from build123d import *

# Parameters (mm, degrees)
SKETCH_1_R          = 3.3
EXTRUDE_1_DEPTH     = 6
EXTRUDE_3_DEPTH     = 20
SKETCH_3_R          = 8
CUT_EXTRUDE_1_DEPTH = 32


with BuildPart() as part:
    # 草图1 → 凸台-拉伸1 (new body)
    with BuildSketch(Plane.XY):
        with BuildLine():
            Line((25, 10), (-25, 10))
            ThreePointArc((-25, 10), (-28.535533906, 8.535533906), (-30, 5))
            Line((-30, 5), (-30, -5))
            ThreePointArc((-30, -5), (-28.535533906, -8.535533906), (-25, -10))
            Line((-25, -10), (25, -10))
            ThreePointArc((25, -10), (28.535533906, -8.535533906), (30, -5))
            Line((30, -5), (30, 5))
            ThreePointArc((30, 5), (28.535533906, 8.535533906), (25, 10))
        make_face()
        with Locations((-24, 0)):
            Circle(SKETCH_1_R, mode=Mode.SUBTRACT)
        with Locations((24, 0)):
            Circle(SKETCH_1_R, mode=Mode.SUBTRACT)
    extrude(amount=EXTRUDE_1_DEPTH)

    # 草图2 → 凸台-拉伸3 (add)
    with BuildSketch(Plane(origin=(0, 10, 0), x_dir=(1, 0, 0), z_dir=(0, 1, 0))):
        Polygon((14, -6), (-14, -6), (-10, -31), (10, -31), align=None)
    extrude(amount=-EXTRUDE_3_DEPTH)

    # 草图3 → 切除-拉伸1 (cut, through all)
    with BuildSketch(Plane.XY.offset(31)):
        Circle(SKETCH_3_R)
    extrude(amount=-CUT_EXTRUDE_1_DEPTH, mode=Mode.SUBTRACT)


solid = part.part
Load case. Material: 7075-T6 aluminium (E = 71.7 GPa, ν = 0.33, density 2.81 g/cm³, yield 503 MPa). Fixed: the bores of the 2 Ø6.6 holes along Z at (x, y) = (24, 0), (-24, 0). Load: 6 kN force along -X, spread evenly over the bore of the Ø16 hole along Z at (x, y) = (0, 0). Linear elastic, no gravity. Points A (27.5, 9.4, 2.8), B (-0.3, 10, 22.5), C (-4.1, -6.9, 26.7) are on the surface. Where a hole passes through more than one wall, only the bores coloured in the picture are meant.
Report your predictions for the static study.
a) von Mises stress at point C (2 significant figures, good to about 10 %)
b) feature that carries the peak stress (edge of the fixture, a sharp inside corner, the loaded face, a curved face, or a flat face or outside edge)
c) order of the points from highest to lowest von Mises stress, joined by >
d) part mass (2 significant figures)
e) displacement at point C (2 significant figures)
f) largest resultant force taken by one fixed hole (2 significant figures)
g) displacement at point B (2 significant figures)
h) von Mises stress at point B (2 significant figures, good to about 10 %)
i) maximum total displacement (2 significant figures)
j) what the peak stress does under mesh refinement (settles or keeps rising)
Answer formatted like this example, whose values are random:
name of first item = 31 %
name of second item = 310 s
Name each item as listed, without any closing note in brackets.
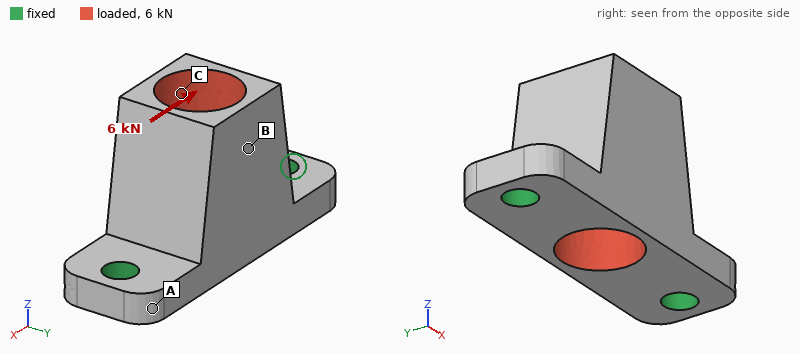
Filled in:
von Mises stress at point C = 23 MPa
feature that carries the peak stress = edge of the fixture
order of the points from highest to lowest von Mises stress, joined by > = B > C > A
part mass = 35 g
displacement at point C = 42 µm
largest resultant force taken by one fixed hole = 3.6 kN
displacement at point B = 35 µm
von Mises stress at point B = 41 MPa
maximum total displacement = 52 µm
what the peak stress does under mesh refinement = keeps rising
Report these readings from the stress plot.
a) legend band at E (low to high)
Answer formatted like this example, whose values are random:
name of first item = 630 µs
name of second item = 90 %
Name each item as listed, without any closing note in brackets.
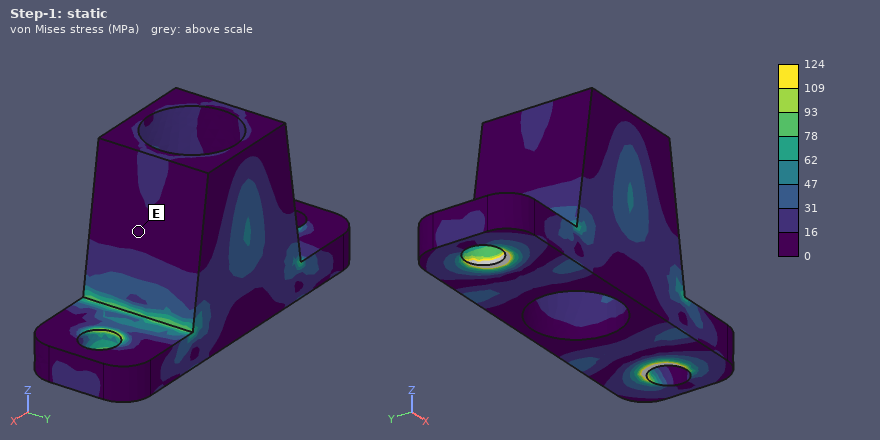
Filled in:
legend band at E = 0 to 16 MPa
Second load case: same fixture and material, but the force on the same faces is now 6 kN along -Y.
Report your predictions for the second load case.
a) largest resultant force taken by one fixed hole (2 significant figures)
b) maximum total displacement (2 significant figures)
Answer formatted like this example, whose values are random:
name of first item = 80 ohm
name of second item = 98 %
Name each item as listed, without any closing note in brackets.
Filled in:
largest resultant force taken by one fixed hole = 3.0 kN
maximum total displacement = 0.34 mm
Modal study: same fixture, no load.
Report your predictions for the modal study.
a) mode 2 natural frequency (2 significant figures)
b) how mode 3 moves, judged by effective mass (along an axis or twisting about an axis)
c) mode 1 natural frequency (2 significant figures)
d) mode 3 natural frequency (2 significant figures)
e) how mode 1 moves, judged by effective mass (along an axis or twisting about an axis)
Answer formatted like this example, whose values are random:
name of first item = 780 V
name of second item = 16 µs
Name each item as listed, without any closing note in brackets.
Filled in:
mode 2 natural frequency = 13 kHz
how mode 3 moves, judged by effective mass = along X
mode 1 natural frequency = 5300 Hz
mode 3 natural frequency = 13 kHz
how mode 1 moves, judged by effective mass = along Y
